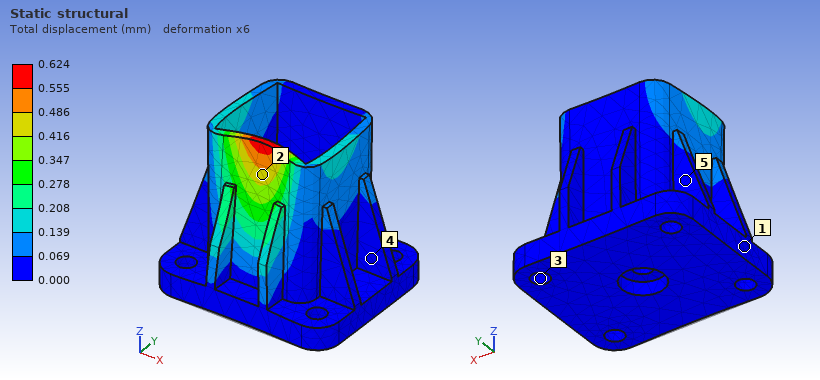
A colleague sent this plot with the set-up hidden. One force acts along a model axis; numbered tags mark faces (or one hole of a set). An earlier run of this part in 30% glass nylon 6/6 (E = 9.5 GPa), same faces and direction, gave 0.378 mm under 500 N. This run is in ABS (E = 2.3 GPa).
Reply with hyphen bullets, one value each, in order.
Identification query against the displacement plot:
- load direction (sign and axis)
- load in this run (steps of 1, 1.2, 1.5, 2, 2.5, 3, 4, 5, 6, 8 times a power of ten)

- +Y
- 200 N
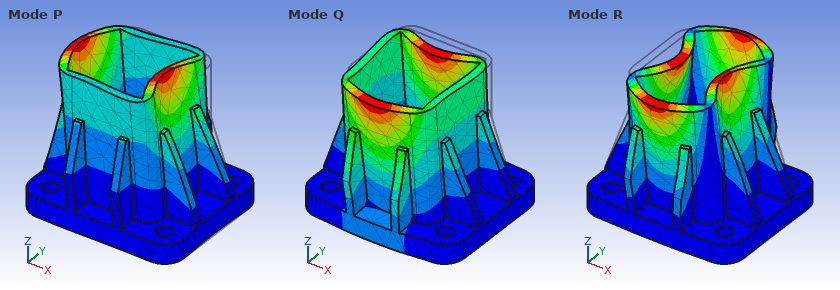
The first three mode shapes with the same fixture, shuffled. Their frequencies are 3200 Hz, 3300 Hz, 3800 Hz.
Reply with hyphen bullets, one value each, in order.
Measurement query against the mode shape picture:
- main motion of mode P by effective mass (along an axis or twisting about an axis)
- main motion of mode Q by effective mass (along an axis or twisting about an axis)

- along X
- along Y
